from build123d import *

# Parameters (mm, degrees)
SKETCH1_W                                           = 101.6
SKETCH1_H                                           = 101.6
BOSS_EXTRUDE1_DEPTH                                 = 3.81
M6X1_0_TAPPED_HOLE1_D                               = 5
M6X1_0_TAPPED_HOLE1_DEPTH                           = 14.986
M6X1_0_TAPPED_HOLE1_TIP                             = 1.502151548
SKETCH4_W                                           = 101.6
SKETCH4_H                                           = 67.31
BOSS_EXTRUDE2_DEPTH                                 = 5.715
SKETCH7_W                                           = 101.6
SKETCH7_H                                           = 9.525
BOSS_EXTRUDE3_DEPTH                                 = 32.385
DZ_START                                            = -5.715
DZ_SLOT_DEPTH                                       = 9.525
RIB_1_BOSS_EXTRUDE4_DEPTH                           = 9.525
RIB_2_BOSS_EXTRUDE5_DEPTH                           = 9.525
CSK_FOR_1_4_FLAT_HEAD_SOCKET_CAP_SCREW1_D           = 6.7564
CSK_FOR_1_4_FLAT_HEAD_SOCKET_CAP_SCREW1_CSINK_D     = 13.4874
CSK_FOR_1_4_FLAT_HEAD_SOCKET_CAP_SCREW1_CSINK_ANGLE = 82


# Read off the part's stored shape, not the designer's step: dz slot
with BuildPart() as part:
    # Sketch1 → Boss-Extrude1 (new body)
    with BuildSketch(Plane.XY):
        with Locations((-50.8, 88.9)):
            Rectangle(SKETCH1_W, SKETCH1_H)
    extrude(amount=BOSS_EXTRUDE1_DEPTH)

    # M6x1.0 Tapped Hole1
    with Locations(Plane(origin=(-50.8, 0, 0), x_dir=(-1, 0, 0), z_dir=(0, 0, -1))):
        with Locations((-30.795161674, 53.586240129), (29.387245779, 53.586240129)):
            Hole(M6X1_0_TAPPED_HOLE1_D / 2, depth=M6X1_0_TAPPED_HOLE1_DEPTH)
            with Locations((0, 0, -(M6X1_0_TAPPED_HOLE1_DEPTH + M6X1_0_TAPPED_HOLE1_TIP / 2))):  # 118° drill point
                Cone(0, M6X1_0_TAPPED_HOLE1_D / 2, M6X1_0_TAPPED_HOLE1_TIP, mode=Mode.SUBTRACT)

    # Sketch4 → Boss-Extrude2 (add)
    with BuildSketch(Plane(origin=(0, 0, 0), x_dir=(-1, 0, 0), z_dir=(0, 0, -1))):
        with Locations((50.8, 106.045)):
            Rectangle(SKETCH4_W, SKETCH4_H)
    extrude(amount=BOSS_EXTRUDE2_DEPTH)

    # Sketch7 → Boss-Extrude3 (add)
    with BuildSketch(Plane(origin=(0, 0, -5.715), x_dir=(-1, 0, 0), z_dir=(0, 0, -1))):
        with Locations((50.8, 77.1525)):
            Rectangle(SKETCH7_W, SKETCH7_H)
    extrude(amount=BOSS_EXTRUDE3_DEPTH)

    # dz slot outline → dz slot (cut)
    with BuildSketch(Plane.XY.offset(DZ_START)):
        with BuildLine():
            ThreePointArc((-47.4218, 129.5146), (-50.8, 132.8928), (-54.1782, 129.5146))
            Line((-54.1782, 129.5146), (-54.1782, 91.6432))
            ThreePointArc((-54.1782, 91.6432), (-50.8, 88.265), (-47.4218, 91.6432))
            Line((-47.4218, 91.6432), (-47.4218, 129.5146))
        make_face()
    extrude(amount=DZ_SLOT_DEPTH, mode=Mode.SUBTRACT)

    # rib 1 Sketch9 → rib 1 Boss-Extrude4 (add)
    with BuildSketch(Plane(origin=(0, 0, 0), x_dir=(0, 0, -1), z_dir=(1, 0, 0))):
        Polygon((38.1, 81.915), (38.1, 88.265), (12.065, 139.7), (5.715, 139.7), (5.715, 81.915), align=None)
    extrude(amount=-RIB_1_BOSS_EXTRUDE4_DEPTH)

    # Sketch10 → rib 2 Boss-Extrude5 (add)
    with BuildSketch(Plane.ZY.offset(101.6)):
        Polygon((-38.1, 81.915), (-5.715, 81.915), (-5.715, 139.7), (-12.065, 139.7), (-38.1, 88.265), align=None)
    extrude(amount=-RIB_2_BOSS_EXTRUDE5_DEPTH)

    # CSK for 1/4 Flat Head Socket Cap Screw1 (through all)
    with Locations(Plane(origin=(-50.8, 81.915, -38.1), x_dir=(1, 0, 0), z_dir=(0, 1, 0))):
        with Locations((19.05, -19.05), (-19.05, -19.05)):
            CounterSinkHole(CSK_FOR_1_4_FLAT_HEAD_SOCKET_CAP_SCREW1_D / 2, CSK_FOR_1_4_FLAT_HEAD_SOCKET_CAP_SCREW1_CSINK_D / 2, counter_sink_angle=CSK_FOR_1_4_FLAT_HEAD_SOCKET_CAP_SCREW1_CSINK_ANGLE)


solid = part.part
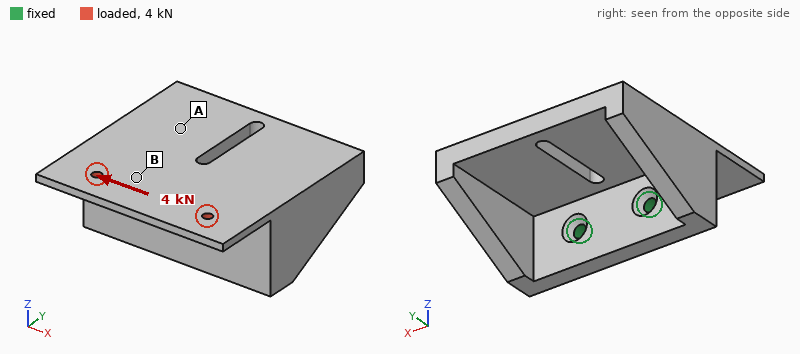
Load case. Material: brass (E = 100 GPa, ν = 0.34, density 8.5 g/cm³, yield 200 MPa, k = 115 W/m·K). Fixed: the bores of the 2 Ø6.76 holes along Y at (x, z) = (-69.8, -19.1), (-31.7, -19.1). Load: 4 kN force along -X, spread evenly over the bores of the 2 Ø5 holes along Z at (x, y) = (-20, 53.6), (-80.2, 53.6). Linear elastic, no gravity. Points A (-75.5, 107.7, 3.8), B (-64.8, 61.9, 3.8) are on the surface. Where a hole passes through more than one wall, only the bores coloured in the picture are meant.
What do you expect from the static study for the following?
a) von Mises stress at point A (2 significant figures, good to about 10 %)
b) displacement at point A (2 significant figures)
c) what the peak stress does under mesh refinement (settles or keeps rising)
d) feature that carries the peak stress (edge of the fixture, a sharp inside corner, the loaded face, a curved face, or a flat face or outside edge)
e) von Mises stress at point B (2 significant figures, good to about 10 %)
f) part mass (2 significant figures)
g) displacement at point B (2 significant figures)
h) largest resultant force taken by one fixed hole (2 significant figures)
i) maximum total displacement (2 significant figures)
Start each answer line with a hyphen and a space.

- 8.7 MPa
- 29 µm
- keeps rising
- edge of the fixture
- 19 MPa
- 1.1 kg
- 24 µm
- 3.3 kN
- 77 µm
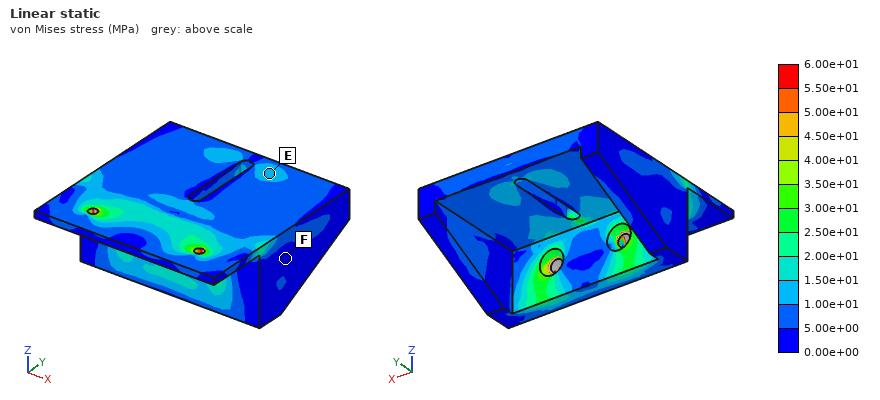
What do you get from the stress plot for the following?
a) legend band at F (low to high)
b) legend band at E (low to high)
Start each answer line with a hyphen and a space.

- 0.00e+00 to 5.00e+00 MPa
- 1.00e+01 to 1.50e+01 MPa
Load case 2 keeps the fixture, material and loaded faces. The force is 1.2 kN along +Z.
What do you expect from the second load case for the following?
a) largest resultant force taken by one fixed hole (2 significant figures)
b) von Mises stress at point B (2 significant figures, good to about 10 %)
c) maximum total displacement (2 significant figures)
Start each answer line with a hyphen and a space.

- 620 N
- 39 MPa
- 0.20 mm
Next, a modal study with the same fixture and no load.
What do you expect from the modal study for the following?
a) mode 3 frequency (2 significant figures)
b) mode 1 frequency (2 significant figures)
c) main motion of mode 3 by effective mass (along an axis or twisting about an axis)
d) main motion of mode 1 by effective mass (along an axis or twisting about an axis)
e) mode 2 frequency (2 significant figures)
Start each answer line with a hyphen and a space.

- 1700 Hz
- 800 Hz
- along Z
- along Z
- 1200 Hz
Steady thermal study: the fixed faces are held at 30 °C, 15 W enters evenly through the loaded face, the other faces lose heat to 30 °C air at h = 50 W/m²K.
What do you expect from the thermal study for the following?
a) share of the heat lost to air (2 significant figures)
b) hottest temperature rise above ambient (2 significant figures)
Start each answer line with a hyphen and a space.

- 35 %
- 13 K
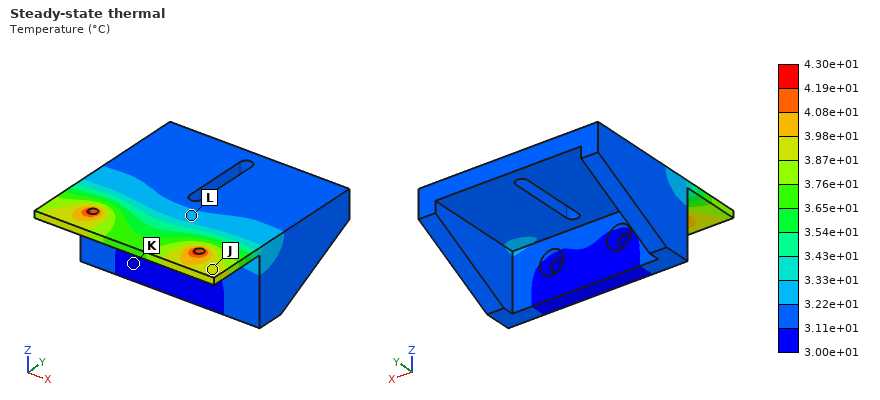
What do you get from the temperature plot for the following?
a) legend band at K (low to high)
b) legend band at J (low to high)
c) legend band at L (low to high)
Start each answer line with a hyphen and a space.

- 3.00e+01 to 3.11e+01 °C
- 3.87e+01 to 3.98e+01 °C
- 3.22e+01 to 3.33e+01 °C
